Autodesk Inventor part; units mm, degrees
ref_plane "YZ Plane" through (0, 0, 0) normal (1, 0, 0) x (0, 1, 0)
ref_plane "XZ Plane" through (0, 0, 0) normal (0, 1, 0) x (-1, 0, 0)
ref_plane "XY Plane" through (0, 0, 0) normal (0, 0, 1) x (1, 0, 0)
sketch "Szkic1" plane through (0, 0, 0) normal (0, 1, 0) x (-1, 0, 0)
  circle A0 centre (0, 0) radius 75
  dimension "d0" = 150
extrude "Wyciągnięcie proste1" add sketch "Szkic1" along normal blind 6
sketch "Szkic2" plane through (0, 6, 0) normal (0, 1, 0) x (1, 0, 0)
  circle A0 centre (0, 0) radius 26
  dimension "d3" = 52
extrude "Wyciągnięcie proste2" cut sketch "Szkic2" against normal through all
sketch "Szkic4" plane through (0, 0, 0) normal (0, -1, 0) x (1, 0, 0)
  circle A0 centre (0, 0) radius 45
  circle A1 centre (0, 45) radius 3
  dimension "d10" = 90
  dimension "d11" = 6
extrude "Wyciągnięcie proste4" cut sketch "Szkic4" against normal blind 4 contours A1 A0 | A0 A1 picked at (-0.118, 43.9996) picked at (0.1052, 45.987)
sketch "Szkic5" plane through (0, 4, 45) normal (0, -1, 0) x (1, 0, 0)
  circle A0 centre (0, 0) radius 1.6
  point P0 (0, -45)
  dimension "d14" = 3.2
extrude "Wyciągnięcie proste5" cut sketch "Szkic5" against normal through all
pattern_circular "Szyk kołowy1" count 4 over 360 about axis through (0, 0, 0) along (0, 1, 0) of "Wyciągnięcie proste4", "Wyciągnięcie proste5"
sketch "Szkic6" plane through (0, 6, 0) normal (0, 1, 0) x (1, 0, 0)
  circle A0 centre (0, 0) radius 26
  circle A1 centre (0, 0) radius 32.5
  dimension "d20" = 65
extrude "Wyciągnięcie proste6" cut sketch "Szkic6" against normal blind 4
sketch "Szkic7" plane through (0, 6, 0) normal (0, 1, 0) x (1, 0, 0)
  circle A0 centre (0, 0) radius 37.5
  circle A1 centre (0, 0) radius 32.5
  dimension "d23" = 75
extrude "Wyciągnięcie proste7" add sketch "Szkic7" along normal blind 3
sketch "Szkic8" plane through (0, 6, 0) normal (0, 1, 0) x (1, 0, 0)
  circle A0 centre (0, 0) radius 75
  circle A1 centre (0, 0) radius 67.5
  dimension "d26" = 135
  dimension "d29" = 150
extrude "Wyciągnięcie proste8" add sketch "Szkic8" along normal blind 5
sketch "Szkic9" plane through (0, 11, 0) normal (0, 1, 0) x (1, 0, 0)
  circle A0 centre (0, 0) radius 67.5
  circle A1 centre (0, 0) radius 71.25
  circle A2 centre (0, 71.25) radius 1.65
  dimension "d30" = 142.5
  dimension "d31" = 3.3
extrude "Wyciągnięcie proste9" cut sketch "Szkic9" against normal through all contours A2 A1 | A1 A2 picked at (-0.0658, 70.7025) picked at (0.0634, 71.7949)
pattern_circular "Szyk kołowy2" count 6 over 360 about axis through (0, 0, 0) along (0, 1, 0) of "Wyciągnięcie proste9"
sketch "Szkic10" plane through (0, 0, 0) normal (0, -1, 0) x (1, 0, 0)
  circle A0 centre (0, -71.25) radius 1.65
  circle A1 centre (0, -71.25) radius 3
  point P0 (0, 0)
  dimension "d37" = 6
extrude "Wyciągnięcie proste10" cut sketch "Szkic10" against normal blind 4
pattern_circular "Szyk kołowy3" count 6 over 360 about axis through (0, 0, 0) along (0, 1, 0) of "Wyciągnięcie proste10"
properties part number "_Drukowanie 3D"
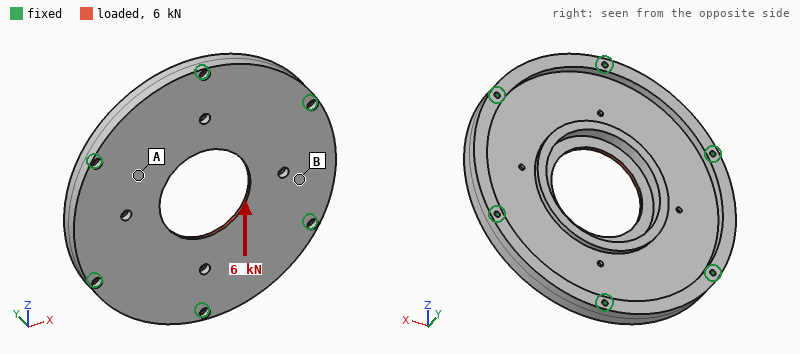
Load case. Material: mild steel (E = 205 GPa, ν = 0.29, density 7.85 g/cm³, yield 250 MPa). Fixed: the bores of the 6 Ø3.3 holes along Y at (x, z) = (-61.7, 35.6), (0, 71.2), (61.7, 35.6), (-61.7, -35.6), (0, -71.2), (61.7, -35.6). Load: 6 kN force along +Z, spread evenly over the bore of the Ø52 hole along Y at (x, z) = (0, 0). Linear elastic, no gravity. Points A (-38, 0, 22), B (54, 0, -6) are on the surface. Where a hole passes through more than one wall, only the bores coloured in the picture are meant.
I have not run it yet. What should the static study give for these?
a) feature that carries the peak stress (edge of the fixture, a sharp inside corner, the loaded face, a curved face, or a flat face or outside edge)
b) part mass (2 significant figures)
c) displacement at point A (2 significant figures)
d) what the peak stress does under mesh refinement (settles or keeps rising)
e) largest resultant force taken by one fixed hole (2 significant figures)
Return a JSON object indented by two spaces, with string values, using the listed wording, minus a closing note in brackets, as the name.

{
  "feature that carries the peak stress": "edge of the fixture",
  "part mass": "840 g",
  "displacement at point A": "2.2 µm",
  "what the peak stress does under mesh refinement": "keeps rising",
  "largest resultant force taken by one fixed hole": "1.2 kN"
}
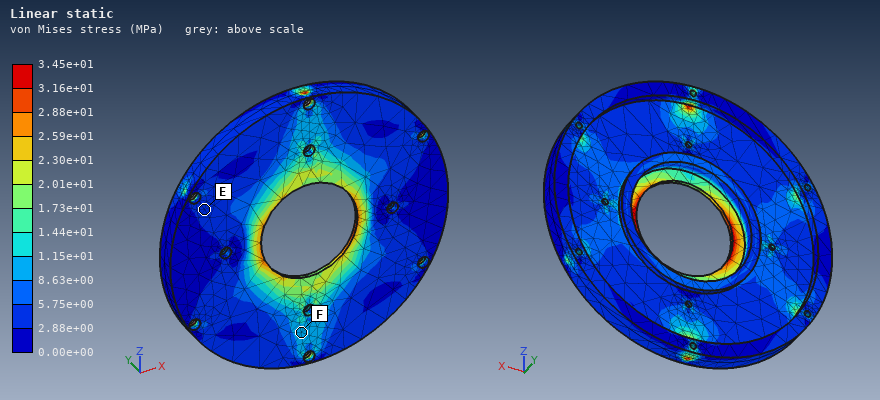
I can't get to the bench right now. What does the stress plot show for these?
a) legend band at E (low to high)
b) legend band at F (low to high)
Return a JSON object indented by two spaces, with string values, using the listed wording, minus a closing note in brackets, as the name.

{
  "legend band at E": "2.88e+00 to 5.75e+00 MPa",
  "legend band at F": "8.63e+00 to 1.15e+01 MPa"
}
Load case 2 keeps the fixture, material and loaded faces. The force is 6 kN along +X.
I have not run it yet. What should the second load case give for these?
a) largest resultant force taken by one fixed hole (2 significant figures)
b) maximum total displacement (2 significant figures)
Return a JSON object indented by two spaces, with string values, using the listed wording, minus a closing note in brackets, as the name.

{
  "largest resultant force taken by one fixed hole": "1.1 kN",
  "maximum total displacement": "7.4 µm"
}
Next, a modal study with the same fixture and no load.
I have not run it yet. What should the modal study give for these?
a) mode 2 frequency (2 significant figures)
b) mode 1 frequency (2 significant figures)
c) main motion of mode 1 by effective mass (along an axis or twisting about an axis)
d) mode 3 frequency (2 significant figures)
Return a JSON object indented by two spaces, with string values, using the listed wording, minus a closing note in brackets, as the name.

{
  "mode 2 frequency": "4300 Hz",
  "mode 1 frequency": "2900 Hz",
  "main motion of mode 1 by effective mass": "along Y",
  "mode 3 frequency": "4300 Hz"
}
